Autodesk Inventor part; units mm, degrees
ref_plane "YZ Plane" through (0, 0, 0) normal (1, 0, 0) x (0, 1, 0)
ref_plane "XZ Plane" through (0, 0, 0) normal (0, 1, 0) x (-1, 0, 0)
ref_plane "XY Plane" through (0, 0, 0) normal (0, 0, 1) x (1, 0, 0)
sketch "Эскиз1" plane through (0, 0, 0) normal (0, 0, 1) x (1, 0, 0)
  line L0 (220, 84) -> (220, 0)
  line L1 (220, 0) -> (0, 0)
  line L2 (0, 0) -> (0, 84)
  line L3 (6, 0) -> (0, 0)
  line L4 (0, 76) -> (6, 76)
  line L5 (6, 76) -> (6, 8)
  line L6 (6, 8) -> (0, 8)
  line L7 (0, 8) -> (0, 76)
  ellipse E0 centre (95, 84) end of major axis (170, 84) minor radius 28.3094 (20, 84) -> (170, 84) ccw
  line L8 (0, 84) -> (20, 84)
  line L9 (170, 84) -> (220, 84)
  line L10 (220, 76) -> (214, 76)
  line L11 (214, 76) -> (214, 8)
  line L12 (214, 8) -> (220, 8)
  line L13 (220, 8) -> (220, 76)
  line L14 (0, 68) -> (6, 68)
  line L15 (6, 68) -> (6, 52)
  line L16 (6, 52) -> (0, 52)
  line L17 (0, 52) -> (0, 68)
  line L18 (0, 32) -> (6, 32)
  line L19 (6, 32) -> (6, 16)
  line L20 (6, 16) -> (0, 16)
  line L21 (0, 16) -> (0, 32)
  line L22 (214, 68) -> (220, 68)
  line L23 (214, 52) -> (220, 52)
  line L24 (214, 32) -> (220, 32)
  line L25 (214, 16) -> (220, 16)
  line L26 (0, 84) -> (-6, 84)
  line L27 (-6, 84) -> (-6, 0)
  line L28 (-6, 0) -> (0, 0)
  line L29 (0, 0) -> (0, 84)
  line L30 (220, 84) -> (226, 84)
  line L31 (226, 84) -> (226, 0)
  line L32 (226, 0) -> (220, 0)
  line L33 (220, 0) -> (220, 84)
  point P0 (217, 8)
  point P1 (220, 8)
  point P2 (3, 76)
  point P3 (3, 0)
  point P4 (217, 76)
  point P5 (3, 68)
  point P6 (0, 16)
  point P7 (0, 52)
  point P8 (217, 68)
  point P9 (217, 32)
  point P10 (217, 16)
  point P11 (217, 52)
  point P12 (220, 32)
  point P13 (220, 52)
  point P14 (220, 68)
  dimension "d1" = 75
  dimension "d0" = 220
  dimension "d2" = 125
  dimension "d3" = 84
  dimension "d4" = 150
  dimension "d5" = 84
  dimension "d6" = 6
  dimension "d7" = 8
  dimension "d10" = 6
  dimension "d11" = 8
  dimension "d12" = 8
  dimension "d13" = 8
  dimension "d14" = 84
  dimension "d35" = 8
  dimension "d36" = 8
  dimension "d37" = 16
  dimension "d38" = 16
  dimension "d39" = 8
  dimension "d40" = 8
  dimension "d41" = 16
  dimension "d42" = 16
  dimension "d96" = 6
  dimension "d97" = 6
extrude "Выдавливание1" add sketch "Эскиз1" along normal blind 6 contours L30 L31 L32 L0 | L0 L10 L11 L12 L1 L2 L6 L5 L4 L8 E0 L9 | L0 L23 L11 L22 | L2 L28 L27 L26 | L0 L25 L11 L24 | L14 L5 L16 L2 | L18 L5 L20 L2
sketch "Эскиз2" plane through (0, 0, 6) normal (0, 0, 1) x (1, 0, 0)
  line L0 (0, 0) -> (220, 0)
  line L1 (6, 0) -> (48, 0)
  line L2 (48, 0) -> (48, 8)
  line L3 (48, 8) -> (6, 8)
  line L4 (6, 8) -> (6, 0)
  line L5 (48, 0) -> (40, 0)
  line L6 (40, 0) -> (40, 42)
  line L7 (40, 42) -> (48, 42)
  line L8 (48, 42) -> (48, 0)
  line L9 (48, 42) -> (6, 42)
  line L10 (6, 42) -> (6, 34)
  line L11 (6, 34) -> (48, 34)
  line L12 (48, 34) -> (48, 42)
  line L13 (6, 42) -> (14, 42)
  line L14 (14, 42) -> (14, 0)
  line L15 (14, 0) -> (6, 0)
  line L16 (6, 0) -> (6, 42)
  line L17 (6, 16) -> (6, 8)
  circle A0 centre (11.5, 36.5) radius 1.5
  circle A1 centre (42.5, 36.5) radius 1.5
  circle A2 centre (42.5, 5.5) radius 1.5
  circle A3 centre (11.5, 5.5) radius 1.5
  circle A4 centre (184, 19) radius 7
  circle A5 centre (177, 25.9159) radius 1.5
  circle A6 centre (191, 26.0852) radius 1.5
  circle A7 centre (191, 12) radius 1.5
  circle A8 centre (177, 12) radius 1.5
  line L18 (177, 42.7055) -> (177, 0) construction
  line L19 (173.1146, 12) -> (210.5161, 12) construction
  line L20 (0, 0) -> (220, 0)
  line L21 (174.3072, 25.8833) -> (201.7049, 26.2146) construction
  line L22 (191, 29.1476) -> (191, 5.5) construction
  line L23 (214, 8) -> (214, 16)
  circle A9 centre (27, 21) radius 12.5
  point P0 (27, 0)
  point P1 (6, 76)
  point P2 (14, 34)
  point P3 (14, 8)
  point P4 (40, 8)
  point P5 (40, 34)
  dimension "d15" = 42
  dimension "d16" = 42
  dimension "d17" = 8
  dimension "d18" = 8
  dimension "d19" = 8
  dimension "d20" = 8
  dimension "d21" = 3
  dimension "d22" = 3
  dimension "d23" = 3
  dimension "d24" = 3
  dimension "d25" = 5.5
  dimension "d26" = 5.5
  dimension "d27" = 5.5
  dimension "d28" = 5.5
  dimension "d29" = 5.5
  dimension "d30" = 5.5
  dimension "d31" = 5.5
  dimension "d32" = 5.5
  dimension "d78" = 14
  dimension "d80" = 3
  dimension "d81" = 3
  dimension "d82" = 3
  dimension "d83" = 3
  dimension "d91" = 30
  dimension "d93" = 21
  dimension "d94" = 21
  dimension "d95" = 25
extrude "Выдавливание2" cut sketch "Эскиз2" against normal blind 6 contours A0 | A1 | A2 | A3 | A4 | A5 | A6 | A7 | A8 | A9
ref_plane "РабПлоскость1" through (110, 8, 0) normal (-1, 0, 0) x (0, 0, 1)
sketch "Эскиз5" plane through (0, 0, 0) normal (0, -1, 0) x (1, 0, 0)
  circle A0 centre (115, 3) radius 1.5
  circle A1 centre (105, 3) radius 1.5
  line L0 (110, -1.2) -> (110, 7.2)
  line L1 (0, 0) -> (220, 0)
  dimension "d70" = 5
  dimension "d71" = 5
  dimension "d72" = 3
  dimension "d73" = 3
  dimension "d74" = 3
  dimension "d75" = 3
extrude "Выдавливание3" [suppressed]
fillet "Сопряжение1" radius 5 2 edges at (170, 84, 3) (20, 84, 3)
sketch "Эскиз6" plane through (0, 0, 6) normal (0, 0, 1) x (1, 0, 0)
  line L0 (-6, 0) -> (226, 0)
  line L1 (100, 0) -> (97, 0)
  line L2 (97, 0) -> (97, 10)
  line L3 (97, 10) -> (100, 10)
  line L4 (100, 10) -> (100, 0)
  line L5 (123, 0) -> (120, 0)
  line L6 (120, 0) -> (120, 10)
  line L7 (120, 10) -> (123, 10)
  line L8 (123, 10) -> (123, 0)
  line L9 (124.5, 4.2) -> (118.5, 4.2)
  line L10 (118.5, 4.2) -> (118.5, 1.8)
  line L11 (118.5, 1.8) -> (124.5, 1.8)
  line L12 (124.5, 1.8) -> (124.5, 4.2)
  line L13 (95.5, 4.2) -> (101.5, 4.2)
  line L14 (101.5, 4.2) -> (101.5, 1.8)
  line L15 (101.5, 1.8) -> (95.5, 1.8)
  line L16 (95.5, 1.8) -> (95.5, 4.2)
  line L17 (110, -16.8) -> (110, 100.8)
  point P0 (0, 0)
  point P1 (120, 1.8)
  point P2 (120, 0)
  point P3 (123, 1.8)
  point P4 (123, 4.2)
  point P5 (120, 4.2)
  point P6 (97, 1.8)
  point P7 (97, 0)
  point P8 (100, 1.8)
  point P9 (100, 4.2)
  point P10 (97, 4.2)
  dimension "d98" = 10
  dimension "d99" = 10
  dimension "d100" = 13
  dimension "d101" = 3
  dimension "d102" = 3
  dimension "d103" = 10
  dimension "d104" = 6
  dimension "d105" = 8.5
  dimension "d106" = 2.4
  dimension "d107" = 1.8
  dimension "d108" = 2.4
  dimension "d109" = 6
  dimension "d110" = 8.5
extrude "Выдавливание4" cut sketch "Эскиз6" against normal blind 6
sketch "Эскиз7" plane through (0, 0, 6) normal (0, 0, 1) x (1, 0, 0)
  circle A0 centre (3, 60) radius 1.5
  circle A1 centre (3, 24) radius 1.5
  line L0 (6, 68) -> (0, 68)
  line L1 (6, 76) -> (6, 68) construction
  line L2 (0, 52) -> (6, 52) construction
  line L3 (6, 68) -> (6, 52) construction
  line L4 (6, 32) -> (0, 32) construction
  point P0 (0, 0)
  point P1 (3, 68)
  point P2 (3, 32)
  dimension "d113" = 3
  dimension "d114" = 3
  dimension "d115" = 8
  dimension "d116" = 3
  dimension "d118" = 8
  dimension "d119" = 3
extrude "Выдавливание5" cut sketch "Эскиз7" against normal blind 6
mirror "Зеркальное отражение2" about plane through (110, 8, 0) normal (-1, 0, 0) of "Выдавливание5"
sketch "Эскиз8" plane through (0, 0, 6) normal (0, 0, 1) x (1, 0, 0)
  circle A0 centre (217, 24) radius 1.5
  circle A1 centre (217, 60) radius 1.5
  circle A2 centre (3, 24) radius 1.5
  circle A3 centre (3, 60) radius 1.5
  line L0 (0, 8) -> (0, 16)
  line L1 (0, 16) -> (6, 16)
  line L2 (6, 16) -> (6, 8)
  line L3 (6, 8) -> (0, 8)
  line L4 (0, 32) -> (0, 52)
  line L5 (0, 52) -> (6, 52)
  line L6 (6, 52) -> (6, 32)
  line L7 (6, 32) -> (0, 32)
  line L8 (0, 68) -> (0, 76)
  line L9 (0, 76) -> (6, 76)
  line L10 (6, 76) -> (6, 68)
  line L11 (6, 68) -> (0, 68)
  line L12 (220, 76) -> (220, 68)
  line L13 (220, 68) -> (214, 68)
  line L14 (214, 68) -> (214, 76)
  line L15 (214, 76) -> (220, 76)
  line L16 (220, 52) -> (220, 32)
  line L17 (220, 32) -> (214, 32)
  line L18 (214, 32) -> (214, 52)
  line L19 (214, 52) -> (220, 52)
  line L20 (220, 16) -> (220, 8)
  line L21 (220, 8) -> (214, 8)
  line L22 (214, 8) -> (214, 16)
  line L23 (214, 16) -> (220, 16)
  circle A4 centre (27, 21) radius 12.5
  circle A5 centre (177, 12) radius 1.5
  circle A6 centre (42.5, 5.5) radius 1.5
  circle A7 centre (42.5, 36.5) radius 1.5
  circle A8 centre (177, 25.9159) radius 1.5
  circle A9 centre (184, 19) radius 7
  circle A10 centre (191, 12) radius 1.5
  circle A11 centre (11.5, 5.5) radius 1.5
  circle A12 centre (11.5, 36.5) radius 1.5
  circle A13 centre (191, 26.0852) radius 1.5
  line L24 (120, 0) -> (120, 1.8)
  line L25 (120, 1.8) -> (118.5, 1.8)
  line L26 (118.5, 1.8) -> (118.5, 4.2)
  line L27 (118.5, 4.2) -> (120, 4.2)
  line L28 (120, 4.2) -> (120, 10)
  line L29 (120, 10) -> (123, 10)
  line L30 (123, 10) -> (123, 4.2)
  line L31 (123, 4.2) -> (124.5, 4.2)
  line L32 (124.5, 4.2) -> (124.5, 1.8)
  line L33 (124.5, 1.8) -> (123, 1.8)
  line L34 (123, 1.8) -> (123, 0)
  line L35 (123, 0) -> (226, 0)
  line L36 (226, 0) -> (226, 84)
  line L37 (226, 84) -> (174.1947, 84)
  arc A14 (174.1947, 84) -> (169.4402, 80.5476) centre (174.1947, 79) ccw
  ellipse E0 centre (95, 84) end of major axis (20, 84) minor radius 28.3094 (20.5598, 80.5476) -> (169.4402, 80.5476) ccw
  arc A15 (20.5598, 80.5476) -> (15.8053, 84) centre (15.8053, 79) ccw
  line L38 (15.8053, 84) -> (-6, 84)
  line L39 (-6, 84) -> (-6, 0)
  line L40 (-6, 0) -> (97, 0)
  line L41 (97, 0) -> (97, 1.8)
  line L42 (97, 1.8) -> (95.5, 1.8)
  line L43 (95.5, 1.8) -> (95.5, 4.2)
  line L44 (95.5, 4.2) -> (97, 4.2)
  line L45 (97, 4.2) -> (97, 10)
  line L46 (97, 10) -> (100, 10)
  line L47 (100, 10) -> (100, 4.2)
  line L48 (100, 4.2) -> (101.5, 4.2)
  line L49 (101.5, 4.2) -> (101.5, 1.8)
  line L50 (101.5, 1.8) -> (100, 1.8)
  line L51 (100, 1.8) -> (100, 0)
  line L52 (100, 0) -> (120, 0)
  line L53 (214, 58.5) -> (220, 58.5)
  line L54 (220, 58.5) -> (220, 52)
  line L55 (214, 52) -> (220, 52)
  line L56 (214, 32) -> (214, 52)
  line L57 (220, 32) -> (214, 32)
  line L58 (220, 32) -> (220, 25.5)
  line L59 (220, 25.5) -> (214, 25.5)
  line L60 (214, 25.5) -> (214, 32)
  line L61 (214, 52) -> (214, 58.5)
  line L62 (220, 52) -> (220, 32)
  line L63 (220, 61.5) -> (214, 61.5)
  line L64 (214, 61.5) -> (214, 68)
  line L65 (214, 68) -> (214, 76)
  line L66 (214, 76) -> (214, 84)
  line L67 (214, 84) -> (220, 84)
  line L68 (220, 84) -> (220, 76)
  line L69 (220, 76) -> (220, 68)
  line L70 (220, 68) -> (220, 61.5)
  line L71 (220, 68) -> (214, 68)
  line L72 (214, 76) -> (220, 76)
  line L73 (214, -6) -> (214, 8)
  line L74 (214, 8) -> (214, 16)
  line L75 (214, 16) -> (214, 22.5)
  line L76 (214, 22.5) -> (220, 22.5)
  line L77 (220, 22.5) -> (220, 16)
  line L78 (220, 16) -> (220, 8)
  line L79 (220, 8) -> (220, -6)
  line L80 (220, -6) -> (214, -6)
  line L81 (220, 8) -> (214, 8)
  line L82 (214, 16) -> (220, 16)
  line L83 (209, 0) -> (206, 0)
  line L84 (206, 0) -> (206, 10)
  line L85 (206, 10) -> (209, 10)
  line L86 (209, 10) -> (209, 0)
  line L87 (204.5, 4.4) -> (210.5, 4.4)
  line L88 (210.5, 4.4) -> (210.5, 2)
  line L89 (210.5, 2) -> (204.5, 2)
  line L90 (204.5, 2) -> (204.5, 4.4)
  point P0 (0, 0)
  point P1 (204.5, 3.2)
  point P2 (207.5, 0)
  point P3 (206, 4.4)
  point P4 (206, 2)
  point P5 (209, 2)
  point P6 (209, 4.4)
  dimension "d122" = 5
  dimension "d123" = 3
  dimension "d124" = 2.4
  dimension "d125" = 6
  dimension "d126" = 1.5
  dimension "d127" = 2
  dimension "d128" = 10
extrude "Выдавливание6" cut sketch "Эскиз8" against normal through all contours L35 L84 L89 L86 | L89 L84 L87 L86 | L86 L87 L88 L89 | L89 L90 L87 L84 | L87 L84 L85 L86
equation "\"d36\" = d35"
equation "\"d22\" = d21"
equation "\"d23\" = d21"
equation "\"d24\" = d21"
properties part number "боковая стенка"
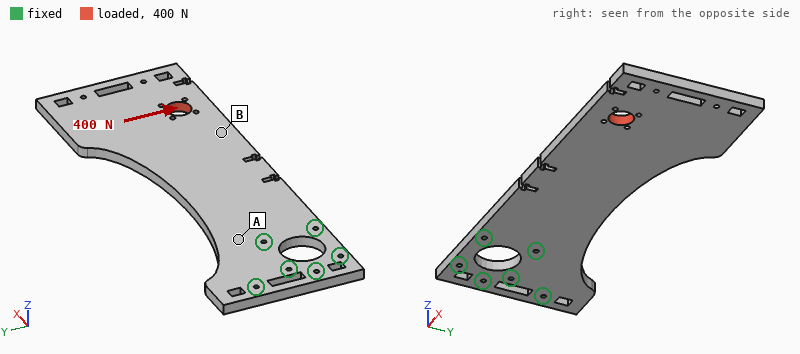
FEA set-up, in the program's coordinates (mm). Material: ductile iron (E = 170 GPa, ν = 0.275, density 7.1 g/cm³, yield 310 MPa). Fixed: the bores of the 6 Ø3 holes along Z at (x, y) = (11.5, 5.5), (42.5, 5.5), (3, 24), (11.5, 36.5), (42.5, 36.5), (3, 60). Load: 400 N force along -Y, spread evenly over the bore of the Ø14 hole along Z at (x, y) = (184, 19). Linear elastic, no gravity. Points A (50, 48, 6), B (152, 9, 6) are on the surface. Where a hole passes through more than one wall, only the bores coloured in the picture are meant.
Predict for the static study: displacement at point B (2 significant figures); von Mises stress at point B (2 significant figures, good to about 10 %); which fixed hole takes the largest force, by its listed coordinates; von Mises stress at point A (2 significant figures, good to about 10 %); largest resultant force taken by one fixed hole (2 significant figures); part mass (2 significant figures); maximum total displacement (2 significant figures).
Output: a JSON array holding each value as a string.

["24 µm", "2.3 MPa", "(42.5, 5.5)", "6.8 MPa", "1.3 kN", "630 g", "52 µm"]
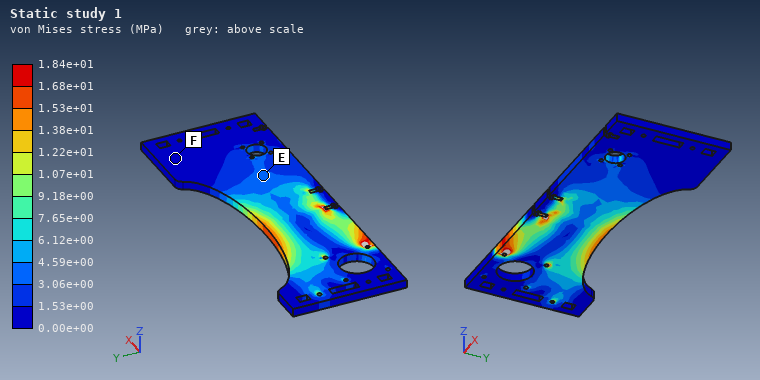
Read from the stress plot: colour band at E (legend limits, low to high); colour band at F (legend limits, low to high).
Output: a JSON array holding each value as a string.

["3.06e+00 to 4.59e+00 MPa", "0.00e+00 to 1.53e+00 MPa"]
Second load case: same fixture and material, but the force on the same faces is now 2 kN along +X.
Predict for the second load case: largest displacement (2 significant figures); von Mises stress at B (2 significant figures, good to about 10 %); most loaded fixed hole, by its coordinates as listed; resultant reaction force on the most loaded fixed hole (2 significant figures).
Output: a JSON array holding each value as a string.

["34 µm", "9.4 MPa", "(42.5, 5.5)", "1.1 kN"]
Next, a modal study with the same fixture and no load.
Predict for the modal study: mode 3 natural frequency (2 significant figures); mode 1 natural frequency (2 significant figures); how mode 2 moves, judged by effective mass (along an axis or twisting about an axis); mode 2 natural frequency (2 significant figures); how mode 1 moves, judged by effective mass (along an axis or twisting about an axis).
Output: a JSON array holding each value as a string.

["830 Hz", "120 Hz", "twisting about X", "570 Hz", "along Z"]
